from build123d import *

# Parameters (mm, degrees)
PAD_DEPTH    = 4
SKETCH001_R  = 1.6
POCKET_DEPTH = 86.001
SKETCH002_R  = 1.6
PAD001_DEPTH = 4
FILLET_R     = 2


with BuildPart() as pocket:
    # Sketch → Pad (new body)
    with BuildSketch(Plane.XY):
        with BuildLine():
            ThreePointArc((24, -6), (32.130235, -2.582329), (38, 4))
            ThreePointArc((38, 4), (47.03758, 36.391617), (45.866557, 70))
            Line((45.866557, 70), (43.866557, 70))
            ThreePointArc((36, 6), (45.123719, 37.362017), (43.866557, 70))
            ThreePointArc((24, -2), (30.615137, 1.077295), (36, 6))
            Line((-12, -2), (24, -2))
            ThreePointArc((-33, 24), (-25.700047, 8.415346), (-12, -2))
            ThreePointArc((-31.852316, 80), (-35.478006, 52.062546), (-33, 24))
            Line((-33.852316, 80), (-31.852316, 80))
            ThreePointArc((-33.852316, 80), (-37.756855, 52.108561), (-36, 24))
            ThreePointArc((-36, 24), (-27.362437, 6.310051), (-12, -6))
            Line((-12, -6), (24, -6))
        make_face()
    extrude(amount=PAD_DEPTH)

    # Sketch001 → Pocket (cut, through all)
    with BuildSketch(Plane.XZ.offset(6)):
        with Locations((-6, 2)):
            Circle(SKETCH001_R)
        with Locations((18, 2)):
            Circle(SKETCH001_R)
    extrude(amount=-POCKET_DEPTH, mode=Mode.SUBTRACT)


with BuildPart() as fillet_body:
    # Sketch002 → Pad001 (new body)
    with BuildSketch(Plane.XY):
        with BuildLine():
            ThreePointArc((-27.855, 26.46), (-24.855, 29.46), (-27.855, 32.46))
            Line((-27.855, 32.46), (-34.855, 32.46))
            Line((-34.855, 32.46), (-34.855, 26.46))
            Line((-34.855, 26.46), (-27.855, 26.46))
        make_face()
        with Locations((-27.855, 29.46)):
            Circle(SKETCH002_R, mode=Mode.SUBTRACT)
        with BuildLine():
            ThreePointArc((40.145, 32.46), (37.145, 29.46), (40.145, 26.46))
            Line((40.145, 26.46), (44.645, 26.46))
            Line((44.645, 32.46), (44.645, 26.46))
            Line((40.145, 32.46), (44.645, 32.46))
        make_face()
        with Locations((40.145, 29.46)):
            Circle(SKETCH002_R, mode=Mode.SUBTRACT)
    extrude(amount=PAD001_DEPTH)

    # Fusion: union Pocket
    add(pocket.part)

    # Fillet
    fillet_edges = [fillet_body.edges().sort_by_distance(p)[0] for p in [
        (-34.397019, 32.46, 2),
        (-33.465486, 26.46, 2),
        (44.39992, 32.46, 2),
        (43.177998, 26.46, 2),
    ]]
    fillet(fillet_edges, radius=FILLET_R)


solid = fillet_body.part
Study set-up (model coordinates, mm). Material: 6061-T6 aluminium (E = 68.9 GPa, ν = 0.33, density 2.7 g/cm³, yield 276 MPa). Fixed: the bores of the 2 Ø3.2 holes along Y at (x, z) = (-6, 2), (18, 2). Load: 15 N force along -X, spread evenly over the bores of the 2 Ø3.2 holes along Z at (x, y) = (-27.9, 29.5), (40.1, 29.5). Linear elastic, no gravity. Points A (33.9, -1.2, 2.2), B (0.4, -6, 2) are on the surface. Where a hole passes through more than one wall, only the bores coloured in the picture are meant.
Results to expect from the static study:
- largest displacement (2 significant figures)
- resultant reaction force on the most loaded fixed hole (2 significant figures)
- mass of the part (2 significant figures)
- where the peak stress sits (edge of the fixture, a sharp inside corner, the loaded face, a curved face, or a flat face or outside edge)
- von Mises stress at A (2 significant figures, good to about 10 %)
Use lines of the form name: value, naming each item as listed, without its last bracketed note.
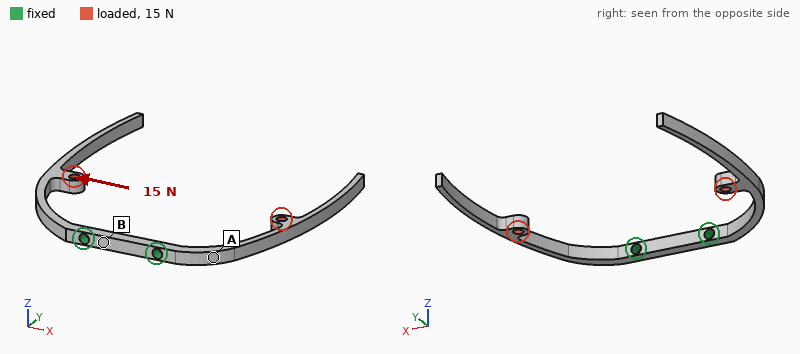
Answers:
largest displacement: 0.90 mm
resultant reaction force on the most loaded fixed hole: 7.5 N
mass of the part: 6.9 g
where the peak stress sits: a curved face
von Mises stress at A: 22 MPa
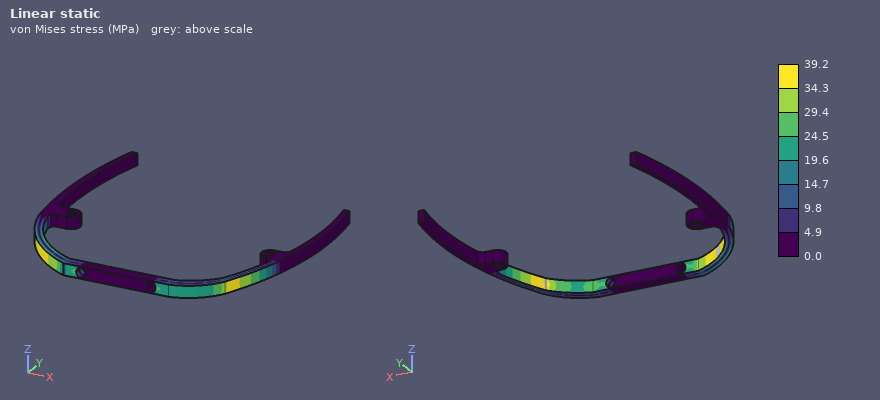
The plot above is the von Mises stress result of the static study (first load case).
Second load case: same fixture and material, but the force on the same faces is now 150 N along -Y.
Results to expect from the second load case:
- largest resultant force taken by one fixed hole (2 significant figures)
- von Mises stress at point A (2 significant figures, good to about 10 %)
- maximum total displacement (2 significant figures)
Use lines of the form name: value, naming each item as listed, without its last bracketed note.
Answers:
largest resultant force taken by one fixed hole: 75 N
von Mises stress at point A: 60 MPa
maximum total displacement: 1.0 mm
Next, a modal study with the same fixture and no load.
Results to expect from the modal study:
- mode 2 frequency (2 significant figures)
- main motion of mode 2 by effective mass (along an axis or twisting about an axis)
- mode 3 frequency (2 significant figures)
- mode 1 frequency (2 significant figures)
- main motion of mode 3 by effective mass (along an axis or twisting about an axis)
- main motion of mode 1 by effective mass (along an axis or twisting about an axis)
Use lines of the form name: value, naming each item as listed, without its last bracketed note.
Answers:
mode 2 frequency: 350 Hz
main motion of mode 2 by effective mass: along Z
mode 3 frequency: 400 Hz
mode 1 frequency: 300 Hz
main motion of mode 3 by effective mass: along X
main motion of mode 1 by effective mass: along X
